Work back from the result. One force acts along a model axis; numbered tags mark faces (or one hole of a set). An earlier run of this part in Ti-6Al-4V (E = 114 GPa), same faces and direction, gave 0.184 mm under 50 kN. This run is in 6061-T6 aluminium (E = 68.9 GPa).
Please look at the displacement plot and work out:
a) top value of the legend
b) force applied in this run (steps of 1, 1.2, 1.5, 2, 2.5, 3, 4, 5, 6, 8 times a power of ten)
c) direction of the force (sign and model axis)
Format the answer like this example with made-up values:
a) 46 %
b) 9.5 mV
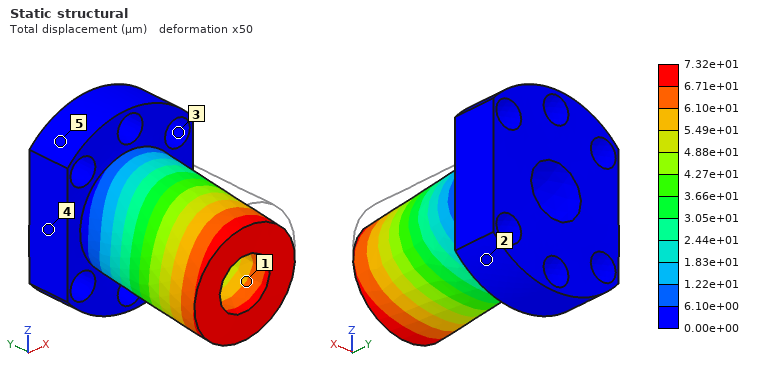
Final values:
a) 7.32e+01 µm
b) 12 kN
c) -Z
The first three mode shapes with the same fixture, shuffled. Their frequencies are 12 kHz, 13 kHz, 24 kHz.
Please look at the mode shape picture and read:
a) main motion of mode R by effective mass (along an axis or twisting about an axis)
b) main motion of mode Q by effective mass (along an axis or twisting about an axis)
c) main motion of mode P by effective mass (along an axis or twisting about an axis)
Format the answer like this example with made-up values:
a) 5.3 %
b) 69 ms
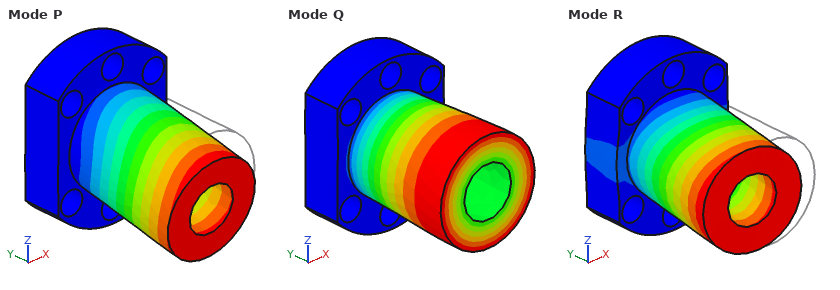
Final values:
a) along X
b) twisting about Y
c) along Z
